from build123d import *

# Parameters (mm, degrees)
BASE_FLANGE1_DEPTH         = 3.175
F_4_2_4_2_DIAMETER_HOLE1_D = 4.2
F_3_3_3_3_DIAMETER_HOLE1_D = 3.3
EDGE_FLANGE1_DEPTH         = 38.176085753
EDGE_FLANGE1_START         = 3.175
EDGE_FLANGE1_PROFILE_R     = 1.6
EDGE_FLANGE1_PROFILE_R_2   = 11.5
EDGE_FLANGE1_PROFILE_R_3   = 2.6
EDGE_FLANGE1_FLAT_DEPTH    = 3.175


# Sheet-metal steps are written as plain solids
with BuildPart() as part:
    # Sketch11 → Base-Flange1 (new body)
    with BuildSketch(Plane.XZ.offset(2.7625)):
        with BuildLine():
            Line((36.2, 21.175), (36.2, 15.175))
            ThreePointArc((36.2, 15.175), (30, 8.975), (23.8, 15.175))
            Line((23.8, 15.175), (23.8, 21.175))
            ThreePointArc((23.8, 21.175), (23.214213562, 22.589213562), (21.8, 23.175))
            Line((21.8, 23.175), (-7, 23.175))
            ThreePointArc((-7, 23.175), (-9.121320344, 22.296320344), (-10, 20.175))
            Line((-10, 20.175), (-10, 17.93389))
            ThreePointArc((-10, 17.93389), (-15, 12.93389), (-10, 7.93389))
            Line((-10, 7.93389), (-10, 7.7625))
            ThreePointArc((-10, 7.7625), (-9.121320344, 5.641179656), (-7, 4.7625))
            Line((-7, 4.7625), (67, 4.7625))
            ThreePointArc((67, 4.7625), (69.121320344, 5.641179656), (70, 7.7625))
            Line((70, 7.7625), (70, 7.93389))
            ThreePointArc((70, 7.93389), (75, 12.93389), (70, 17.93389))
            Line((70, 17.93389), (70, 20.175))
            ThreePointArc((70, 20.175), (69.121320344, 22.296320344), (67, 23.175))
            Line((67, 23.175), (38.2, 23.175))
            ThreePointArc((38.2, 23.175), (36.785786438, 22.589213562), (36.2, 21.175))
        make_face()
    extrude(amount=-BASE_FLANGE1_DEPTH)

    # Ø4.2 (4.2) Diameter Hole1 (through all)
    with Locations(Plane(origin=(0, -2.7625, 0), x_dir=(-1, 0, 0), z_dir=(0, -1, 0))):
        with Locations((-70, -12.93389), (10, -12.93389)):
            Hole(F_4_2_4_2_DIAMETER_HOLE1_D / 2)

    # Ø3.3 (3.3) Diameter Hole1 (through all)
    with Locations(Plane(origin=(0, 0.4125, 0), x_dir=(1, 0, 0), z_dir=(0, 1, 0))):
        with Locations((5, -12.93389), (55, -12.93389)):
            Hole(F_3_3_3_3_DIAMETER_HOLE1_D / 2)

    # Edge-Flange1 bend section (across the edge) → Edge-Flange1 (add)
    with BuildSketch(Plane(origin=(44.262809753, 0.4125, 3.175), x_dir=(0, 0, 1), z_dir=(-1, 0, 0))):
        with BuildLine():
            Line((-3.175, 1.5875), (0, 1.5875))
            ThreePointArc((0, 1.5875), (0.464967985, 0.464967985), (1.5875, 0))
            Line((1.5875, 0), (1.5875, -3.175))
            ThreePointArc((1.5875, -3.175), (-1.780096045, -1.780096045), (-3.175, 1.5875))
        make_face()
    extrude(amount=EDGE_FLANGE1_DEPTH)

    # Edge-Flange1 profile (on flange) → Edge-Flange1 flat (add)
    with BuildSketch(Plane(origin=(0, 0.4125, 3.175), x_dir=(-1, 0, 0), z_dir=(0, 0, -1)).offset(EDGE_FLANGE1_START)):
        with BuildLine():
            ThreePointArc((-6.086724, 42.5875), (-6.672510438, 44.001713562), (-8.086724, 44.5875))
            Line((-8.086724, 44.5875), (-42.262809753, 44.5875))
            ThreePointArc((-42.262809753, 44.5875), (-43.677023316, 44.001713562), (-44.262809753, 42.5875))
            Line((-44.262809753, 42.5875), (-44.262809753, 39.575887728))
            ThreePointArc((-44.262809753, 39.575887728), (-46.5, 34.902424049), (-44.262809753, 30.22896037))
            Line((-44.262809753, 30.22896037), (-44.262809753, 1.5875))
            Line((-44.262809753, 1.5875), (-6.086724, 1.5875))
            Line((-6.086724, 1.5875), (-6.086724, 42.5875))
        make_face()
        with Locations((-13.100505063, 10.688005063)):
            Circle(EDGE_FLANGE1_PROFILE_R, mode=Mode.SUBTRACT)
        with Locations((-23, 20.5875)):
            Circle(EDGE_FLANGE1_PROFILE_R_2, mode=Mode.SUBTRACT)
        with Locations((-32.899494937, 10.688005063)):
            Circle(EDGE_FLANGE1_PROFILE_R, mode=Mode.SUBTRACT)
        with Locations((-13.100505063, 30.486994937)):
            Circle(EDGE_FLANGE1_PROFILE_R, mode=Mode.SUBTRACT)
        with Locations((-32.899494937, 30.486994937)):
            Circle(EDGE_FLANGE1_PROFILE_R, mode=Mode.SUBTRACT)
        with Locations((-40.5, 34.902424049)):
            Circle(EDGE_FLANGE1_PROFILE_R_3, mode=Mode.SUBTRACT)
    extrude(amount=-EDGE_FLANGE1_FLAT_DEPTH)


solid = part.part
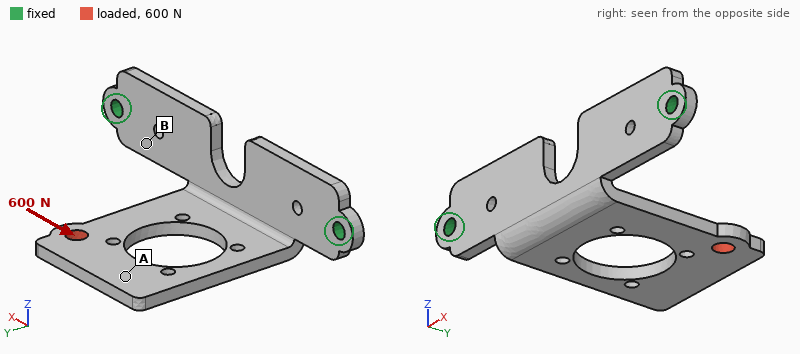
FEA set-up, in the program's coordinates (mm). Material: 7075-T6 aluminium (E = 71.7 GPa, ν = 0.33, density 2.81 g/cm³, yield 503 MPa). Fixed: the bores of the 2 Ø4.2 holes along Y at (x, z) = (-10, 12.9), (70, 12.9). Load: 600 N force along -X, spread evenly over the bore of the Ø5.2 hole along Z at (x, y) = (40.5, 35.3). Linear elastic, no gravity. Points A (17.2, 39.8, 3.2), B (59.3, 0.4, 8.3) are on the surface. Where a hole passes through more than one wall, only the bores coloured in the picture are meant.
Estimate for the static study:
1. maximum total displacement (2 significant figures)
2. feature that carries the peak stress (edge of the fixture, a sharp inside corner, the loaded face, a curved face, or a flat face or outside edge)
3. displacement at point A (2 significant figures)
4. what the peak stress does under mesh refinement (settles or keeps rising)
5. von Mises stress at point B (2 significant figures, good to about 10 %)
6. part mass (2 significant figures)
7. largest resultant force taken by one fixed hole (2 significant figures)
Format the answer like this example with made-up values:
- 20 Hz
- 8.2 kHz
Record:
- 0.84 mm
- a sharp inside corner
- 0.64 mm
- keeps rising
- 89 MPa
- 24 g
- 510 N
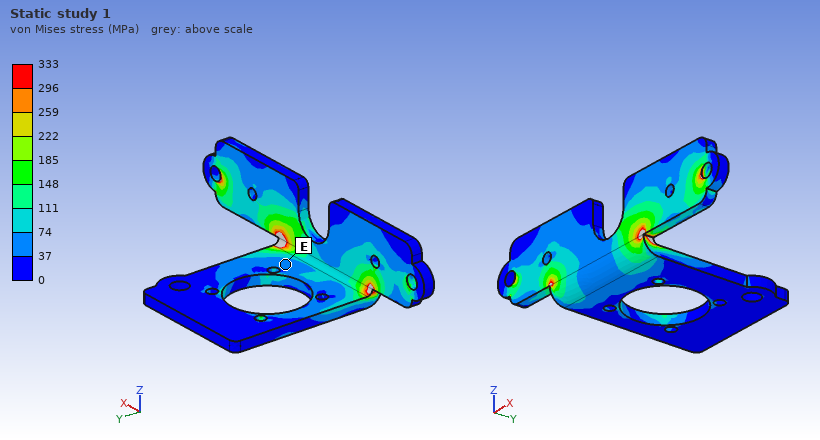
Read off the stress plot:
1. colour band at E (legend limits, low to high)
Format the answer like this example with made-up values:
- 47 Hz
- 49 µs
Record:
- 37 to 74 MPa
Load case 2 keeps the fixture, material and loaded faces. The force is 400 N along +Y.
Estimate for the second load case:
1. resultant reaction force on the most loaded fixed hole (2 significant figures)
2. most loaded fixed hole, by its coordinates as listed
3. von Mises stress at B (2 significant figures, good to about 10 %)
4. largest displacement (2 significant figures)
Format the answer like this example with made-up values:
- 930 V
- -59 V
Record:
- 280 N
- (70, 12.9)
- 100 MPa
- 0.81 mm
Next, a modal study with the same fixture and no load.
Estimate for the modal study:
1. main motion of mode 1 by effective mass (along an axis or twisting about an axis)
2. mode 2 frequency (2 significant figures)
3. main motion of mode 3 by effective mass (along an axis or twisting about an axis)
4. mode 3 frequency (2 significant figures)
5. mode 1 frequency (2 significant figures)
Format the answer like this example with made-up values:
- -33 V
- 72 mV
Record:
- along Z
- 1600 Hz
- along Y
- 2200 Hz
- 650 Hz
